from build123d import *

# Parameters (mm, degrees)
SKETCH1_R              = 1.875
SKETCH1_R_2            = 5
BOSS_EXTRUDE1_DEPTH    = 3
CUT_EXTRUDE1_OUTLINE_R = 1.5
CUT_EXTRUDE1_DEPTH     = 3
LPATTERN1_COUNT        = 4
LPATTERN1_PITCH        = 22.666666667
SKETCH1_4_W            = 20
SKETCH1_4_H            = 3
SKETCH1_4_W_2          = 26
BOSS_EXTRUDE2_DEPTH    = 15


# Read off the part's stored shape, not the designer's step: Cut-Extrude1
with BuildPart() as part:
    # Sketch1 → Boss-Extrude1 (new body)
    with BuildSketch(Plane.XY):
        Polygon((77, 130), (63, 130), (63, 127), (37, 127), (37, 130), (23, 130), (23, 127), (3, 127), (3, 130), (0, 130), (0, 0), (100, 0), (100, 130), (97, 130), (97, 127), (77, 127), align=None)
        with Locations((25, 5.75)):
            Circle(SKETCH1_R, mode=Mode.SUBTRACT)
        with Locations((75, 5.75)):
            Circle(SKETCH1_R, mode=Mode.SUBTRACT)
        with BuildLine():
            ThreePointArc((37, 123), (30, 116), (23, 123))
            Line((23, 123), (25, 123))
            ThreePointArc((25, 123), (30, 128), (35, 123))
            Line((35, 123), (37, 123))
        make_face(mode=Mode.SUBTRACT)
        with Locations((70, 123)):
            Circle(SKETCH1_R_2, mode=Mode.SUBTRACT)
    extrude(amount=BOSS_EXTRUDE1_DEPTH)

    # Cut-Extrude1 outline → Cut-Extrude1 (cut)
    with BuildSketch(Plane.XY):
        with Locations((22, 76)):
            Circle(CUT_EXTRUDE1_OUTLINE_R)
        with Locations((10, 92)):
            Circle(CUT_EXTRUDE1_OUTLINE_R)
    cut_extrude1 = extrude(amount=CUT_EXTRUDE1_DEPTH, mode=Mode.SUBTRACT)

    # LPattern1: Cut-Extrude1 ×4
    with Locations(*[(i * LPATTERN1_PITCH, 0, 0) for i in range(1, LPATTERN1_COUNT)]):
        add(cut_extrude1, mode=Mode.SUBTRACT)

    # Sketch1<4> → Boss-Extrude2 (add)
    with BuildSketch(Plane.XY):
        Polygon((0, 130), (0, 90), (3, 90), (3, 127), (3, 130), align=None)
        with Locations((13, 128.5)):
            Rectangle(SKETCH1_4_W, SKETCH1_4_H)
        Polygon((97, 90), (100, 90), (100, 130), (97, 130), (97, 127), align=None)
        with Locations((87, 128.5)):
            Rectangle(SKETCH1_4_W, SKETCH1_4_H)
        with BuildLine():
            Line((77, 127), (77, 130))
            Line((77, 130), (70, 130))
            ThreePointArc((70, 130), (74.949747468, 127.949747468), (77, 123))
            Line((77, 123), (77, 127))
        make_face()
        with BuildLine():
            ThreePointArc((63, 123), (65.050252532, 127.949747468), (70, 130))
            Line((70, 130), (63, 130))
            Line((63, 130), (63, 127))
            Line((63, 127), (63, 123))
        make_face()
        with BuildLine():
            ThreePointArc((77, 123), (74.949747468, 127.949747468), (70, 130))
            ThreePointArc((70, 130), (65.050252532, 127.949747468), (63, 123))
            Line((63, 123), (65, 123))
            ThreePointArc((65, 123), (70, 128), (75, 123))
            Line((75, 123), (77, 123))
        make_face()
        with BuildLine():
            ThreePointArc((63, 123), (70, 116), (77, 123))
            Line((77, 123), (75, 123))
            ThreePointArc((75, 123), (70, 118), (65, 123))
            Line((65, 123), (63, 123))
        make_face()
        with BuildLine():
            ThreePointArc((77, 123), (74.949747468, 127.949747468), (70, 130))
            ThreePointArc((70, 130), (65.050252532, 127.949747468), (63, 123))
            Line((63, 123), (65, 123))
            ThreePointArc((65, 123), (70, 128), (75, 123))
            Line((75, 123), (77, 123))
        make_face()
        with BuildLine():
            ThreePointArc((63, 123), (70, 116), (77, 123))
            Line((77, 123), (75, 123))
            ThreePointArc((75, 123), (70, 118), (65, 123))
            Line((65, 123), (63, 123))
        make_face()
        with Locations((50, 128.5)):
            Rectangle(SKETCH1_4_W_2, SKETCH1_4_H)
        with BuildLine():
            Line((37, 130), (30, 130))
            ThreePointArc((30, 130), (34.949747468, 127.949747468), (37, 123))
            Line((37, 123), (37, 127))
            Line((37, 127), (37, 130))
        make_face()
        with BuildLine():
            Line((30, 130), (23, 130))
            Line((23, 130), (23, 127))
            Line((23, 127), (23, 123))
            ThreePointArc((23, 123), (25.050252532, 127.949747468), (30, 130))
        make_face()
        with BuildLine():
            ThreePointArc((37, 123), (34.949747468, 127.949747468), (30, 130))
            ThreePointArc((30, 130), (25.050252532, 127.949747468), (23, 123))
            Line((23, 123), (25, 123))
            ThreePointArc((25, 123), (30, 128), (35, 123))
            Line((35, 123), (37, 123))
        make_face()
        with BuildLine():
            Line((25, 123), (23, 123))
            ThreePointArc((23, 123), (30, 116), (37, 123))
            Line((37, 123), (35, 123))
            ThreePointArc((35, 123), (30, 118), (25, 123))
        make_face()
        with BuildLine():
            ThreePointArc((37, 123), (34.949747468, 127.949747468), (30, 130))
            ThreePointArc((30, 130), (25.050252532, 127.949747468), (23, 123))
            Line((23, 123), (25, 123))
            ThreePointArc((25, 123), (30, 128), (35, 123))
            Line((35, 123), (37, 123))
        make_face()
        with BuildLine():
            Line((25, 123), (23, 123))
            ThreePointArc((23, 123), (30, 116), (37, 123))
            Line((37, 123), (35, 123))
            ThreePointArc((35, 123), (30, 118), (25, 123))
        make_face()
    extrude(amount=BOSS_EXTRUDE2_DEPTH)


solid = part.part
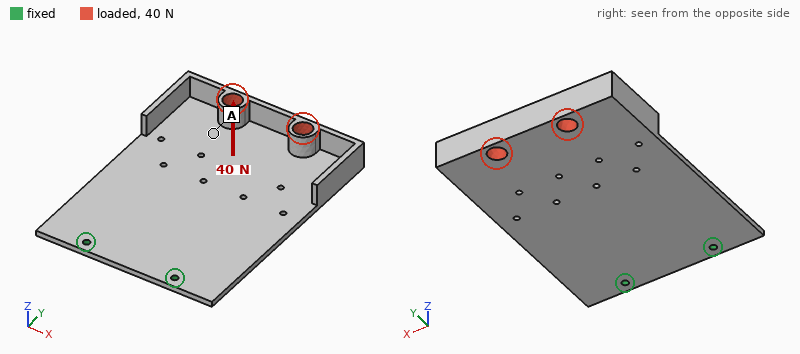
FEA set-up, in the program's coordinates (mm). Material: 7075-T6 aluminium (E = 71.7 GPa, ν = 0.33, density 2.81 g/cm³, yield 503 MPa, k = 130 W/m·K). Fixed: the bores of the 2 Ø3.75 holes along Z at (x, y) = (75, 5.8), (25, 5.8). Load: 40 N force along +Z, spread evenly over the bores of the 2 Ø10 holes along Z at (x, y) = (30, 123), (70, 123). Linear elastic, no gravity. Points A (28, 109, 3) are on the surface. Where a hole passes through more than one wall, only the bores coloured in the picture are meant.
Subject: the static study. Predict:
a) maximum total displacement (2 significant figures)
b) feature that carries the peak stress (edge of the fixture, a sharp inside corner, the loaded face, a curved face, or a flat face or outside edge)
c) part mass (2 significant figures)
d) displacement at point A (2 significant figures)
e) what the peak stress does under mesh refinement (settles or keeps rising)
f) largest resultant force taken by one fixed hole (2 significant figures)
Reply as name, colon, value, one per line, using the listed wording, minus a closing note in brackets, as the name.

maximum total displacement: 1.6 mm
feature that carries the peak stress: edge of the fixture
part mass: 130 g
displacement at point A: 1.2 mm
what the peak stress does under mesh refinement: keeps rising
largest resultant force taken by one fixed hole: 20 N
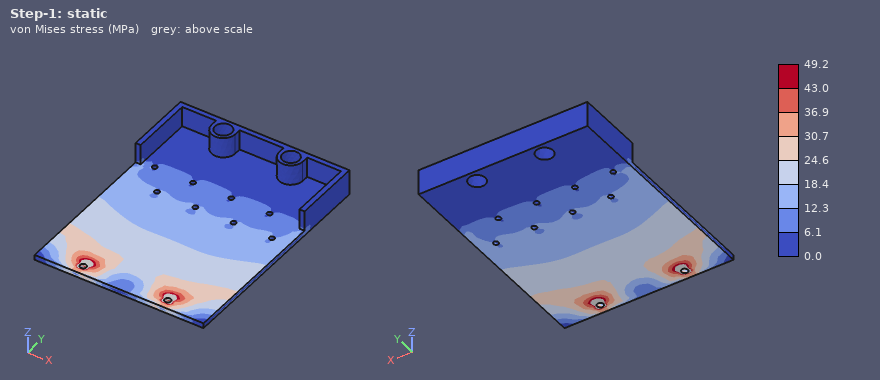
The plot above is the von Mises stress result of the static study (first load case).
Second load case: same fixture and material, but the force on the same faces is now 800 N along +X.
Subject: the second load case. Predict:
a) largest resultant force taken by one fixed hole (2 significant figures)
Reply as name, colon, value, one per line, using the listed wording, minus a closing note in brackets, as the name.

largest resultant force taken by one fixed hole: 1.9 kN
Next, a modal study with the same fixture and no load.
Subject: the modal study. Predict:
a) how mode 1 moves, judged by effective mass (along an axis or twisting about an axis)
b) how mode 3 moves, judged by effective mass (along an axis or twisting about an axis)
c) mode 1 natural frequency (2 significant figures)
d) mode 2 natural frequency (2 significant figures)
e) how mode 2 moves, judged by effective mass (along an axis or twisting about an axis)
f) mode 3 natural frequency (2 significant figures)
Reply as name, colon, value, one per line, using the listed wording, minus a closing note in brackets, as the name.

how mode 1 moves, judged by effective mass: along Z
how mode 3 moves, judged by effective mass: along Z
mode 1 natural frequency: 120 Hz
mode 2 natural frequency: 350 Hz
how mode 2 moves, judged by effective mass: twisting about Y
mode 3 natural frequency: 820 Hz
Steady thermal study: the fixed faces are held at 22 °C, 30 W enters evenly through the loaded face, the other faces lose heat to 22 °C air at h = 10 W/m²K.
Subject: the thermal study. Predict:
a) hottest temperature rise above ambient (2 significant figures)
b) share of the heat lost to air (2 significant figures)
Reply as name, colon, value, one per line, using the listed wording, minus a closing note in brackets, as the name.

hottest temperature rise above ambient: 75 K
share of the heat lost to air: 42 %
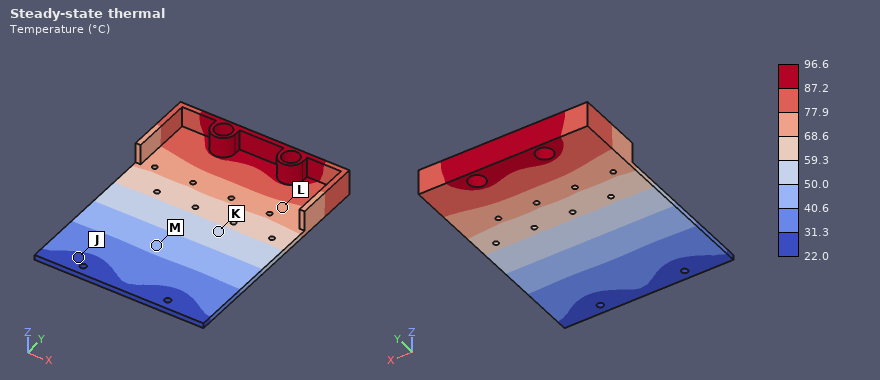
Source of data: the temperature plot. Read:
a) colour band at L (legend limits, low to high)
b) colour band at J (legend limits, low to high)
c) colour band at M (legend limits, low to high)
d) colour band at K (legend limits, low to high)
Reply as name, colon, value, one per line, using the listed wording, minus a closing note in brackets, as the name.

colour band at L: 68.6 to 77.9 °C
colour band at J: 22.0 to 31.3 °C
colour band at M: 40.6 to 50.0 °C
colour band at K: 50.0 to 59.3 °C
